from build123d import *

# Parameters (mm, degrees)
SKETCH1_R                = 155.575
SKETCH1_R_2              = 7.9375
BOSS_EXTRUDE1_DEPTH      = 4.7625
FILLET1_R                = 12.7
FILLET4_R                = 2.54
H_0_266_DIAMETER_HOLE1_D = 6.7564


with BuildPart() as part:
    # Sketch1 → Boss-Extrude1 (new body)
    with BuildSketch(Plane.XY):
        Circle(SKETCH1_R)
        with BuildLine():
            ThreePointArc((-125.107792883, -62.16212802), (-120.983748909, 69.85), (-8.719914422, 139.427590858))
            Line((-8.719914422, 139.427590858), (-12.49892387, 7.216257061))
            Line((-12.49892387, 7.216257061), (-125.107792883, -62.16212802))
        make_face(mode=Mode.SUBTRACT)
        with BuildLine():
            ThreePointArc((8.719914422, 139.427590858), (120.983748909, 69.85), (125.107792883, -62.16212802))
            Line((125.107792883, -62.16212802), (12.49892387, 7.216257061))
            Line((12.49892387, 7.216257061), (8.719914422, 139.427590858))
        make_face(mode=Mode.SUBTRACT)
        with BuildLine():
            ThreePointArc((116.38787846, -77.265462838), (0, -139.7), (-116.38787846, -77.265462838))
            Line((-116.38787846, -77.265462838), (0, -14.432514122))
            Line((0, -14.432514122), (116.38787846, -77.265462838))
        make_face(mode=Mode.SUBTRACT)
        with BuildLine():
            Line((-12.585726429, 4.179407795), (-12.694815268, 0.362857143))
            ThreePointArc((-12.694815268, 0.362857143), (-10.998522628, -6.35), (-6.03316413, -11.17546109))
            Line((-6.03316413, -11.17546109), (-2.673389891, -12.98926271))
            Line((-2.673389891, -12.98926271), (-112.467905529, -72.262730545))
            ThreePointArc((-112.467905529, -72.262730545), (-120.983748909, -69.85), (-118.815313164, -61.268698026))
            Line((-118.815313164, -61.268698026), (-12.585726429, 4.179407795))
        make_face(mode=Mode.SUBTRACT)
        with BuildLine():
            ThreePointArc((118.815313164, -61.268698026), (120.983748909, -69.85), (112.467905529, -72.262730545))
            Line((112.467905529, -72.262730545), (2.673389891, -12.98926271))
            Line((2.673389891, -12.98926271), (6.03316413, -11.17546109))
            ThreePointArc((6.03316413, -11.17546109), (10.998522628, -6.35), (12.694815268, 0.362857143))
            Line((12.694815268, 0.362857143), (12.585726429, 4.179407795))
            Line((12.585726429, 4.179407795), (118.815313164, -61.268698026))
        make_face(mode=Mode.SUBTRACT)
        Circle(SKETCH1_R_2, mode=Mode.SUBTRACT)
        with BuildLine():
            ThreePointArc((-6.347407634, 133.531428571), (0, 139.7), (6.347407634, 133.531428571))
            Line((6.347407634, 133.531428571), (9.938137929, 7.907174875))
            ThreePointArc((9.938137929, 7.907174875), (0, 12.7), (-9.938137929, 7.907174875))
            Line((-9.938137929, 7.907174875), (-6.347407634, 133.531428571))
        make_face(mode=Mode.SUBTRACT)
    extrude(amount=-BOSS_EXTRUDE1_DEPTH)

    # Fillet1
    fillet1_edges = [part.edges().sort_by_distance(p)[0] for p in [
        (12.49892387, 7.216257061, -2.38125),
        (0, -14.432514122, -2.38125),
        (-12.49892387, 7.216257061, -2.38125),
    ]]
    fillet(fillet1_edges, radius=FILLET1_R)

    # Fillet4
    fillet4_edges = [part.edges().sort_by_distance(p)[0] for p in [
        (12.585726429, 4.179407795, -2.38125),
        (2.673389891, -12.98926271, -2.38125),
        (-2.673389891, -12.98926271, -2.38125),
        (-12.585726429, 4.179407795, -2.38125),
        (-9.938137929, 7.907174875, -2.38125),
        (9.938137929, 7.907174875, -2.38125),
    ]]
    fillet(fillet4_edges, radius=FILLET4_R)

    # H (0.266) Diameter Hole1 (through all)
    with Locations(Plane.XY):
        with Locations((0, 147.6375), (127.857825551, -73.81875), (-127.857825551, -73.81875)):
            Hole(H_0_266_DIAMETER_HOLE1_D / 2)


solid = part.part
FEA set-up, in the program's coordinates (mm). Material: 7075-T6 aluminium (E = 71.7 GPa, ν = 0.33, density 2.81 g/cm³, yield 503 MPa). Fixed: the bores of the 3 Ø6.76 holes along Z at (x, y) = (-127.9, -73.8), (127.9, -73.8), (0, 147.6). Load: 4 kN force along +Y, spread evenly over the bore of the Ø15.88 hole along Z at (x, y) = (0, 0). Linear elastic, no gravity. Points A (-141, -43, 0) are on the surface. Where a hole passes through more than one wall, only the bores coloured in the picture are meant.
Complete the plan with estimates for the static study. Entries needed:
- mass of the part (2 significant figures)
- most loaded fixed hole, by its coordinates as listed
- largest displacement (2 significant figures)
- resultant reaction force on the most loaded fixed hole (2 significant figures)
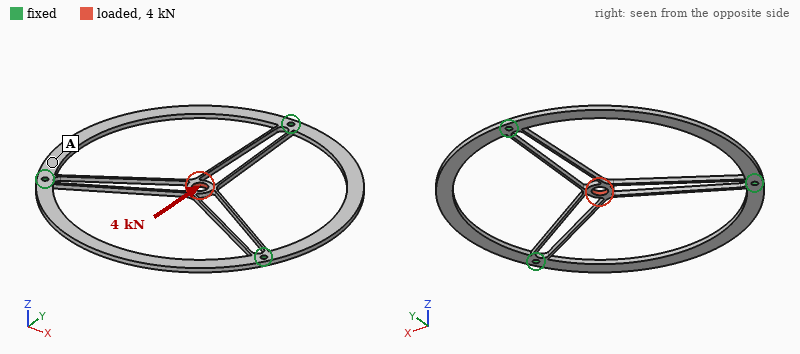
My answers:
230 g
(0, 147.6)
0.22 mm
2.6 kN
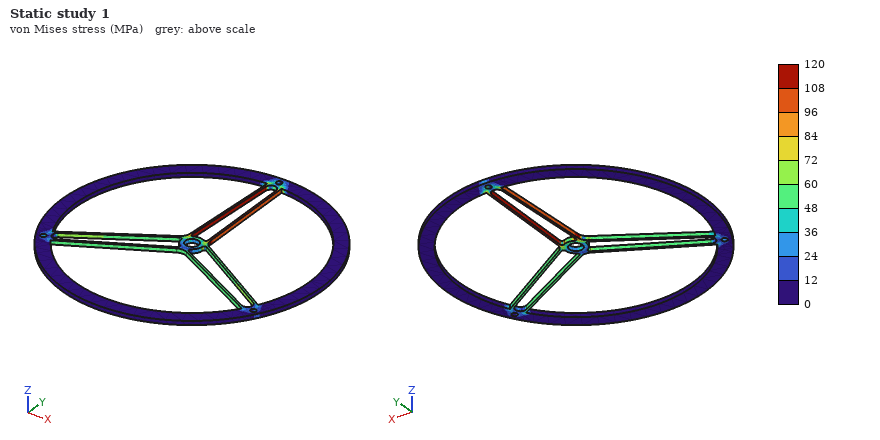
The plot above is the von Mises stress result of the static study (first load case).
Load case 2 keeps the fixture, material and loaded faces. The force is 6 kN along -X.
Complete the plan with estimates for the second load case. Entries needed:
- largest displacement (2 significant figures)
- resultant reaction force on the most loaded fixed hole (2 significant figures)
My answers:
0.33 mm
3.4 kN
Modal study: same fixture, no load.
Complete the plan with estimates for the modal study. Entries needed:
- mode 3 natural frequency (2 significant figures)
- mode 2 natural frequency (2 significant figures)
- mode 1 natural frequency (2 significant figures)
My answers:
240 Hz
240 Hz
240 Hz
